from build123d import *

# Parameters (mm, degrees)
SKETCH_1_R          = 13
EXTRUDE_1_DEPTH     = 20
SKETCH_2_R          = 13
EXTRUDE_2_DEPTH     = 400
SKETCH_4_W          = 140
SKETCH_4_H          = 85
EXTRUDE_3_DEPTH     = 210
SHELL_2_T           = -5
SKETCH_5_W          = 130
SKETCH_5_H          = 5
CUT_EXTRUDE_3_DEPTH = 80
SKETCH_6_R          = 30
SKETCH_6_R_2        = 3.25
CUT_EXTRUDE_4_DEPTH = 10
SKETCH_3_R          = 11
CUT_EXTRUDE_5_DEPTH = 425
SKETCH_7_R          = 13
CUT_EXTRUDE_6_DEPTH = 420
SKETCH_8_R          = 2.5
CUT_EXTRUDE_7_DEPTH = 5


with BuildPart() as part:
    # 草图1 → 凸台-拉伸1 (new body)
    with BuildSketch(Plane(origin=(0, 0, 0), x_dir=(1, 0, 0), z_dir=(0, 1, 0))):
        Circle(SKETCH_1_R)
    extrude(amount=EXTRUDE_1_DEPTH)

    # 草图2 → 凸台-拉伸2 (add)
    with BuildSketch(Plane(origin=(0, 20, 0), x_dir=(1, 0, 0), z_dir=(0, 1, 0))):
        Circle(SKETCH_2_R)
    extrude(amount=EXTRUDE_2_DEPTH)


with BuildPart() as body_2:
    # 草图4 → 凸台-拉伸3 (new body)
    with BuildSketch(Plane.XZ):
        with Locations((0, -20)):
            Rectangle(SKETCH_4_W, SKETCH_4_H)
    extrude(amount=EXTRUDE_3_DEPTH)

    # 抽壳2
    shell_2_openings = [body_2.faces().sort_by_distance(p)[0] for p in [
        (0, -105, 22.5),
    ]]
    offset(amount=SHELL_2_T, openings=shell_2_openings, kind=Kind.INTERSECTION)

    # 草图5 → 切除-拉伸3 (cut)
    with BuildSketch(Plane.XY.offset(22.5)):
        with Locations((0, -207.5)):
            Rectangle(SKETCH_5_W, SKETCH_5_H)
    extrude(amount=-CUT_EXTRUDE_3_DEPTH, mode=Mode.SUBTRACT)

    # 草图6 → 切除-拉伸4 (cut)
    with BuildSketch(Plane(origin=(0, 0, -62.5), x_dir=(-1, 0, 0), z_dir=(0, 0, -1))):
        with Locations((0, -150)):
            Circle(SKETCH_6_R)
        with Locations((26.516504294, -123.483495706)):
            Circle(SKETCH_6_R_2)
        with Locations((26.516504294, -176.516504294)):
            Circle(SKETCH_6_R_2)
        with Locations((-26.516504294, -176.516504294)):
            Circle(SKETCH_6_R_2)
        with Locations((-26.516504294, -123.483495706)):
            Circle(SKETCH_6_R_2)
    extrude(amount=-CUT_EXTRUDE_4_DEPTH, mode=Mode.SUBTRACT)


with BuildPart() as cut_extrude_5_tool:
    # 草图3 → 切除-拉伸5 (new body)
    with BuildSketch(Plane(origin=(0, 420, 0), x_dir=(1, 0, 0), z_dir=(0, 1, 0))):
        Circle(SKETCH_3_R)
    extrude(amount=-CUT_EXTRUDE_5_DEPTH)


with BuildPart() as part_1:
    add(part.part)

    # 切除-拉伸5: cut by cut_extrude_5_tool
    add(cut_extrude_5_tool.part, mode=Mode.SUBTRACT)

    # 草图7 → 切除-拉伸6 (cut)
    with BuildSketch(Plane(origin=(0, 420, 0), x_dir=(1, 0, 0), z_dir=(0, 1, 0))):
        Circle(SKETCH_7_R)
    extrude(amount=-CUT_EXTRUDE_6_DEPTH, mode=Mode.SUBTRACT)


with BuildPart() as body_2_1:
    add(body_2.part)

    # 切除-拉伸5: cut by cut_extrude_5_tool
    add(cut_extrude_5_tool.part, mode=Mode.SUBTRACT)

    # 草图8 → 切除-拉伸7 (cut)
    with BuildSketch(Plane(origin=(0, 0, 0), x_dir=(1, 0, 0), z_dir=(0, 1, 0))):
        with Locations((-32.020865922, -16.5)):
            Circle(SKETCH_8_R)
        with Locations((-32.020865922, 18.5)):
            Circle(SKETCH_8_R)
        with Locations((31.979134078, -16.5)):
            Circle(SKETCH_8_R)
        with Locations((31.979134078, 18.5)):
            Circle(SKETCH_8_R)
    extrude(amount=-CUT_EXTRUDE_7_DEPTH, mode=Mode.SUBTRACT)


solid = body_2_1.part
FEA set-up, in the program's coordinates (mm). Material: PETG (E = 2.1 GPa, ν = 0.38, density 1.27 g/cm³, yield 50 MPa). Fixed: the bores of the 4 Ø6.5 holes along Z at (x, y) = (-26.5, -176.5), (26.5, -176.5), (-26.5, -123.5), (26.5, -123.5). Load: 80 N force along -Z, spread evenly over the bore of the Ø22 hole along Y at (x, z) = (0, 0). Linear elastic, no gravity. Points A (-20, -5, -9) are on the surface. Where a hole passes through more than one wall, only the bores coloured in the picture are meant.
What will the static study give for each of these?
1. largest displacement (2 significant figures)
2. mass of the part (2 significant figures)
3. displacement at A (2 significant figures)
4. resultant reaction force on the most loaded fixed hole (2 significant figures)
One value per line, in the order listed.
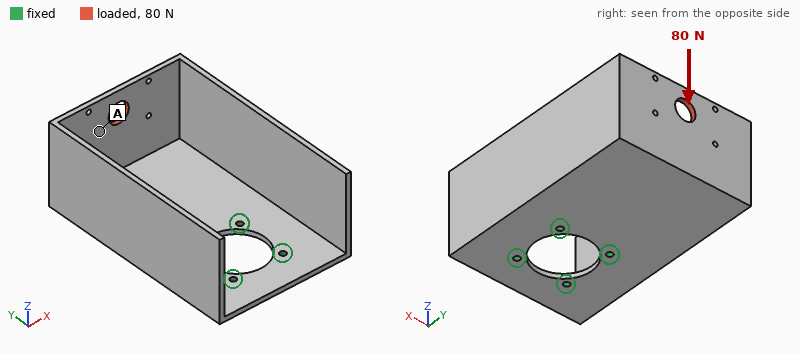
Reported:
2.9 mm
440 g
2.6 mm
99 N
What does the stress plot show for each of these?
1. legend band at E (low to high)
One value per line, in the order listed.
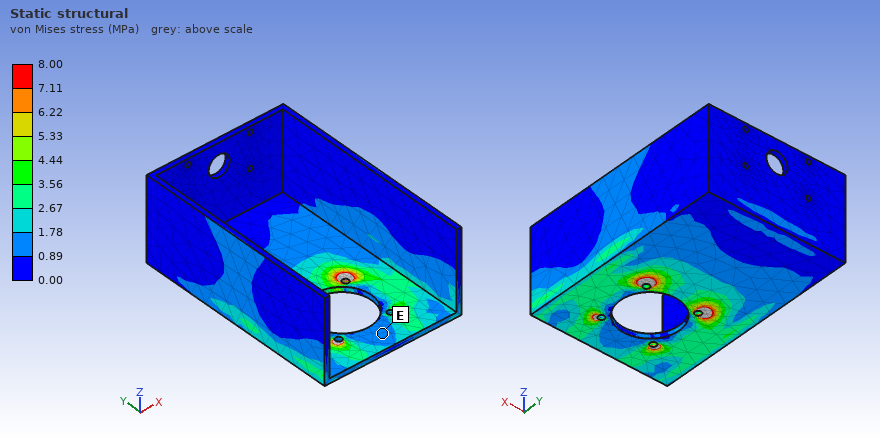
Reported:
0.89 to 1.78 MPa
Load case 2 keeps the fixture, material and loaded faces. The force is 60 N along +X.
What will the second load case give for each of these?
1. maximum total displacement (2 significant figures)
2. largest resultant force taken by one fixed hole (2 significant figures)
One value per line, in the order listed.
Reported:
2.6 mm
99 N
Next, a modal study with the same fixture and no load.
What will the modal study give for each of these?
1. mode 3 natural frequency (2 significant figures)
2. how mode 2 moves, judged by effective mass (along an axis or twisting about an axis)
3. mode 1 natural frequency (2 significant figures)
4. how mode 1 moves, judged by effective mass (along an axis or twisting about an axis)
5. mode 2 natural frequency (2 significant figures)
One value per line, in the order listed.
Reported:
100 Hz
along Z
63 Hz
along X
65 Hz
